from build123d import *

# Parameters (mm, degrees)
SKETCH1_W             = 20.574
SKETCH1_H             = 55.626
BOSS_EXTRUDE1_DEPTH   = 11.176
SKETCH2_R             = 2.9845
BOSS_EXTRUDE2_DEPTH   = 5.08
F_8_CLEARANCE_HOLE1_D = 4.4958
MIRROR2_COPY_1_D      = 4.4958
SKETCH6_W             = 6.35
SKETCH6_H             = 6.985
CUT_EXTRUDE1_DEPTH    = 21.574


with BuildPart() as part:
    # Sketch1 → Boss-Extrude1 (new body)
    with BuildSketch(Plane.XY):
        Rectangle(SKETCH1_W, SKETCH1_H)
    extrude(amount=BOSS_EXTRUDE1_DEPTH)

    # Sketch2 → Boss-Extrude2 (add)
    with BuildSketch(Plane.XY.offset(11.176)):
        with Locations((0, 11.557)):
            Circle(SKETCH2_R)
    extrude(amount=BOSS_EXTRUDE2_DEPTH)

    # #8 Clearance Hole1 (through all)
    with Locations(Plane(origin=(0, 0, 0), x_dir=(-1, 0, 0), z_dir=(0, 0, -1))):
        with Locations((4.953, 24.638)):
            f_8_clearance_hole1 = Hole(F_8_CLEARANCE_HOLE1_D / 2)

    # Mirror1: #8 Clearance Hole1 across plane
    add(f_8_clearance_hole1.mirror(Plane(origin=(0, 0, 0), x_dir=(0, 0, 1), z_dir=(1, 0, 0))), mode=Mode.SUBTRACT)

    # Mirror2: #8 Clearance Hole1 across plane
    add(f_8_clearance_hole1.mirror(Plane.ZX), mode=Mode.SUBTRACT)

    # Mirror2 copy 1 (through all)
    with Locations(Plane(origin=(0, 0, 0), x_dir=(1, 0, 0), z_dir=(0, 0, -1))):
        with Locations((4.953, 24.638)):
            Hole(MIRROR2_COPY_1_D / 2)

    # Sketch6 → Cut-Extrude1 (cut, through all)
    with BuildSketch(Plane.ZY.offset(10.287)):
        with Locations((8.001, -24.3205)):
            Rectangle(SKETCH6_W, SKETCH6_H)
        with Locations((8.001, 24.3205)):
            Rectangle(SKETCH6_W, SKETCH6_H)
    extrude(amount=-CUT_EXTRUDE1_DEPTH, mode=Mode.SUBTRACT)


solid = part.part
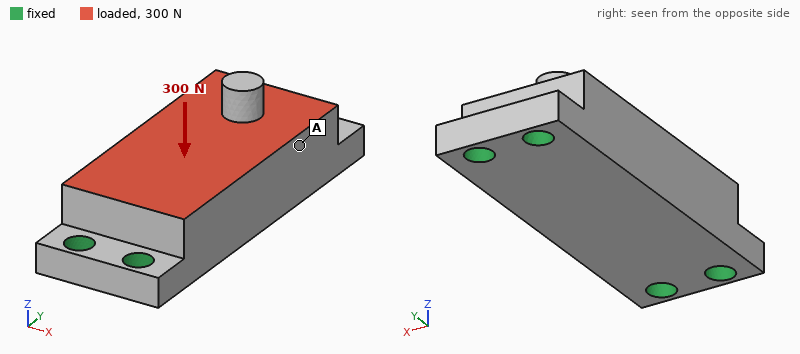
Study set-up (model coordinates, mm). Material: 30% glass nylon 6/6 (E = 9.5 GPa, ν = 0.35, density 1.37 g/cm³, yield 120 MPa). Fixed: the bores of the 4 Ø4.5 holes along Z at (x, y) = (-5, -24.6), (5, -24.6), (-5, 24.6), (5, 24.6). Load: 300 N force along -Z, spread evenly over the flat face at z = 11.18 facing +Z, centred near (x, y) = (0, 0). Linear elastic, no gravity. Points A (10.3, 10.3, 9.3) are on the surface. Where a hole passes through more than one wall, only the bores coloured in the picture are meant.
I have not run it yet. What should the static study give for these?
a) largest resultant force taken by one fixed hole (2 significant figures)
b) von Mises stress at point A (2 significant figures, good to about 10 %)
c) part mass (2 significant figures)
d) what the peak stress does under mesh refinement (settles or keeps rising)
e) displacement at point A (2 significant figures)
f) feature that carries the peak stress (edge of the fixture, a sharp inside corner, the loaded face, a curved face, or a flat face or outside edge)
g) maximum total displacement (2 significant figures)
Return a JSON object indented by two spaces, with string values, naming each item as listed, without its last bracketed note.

{
  "largest resultant force taken by one fixed hole": "100 N",
  "von Mises stress at point A": "1.5 MPa",
  "part mass": "15 g",
  "what the peak stress does under mesh refinement": "keeps rising",
  "displacement at point A": "9.4 µm",
  "feature that carries the peak stress": "edge of the fixture",
  "maximum total displacement": "12 µm"
}
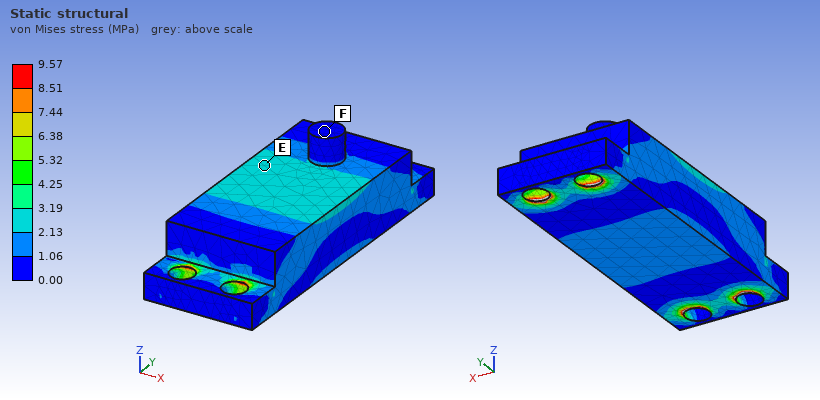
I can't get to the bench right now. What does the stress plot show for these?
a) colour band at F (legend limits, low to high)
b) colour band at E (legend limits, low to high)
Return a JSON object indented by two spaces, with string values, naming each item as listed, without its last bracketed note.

{
  "colour band at F": "0.00 to 1.06 MPa",
  "colour band at E": "2.13 to 3.19 MPa"
}
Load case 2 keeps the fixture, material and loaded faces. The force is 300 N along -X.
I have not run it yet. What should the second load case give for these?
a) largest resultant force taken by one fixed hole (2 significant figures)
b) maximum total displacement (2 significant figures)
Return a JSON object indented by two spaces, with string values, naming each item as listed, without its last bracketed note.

{
  "largest resultant force taken by one fixed hole": "150 N",
  "maximum total displacement": "19 µm"
}
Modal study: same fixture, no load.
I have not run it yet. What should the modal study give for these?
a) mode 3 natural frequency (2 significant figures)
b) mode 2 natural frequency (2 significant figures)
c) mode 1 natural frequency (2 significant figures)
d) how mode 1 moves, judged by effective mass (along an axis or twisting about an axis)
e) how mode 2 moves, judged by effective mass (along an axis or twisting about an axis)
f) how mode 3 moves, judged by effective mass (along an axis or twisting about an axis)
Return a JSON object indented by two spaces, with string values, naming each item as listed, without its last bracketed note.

{
  "mode 3 natural frequency": "11 kHz",
  "mode 2 natural frequency": "8700 Hz",
  "mode 1 natural frequency": "7600 Hz",
  "how mode 1 moves, judged by effective mass": "along Z",
  "how mode 2 moves, judged by effective mass": "along X",
  "how mode 3 moves, judged by effective mass": "along X"
}
